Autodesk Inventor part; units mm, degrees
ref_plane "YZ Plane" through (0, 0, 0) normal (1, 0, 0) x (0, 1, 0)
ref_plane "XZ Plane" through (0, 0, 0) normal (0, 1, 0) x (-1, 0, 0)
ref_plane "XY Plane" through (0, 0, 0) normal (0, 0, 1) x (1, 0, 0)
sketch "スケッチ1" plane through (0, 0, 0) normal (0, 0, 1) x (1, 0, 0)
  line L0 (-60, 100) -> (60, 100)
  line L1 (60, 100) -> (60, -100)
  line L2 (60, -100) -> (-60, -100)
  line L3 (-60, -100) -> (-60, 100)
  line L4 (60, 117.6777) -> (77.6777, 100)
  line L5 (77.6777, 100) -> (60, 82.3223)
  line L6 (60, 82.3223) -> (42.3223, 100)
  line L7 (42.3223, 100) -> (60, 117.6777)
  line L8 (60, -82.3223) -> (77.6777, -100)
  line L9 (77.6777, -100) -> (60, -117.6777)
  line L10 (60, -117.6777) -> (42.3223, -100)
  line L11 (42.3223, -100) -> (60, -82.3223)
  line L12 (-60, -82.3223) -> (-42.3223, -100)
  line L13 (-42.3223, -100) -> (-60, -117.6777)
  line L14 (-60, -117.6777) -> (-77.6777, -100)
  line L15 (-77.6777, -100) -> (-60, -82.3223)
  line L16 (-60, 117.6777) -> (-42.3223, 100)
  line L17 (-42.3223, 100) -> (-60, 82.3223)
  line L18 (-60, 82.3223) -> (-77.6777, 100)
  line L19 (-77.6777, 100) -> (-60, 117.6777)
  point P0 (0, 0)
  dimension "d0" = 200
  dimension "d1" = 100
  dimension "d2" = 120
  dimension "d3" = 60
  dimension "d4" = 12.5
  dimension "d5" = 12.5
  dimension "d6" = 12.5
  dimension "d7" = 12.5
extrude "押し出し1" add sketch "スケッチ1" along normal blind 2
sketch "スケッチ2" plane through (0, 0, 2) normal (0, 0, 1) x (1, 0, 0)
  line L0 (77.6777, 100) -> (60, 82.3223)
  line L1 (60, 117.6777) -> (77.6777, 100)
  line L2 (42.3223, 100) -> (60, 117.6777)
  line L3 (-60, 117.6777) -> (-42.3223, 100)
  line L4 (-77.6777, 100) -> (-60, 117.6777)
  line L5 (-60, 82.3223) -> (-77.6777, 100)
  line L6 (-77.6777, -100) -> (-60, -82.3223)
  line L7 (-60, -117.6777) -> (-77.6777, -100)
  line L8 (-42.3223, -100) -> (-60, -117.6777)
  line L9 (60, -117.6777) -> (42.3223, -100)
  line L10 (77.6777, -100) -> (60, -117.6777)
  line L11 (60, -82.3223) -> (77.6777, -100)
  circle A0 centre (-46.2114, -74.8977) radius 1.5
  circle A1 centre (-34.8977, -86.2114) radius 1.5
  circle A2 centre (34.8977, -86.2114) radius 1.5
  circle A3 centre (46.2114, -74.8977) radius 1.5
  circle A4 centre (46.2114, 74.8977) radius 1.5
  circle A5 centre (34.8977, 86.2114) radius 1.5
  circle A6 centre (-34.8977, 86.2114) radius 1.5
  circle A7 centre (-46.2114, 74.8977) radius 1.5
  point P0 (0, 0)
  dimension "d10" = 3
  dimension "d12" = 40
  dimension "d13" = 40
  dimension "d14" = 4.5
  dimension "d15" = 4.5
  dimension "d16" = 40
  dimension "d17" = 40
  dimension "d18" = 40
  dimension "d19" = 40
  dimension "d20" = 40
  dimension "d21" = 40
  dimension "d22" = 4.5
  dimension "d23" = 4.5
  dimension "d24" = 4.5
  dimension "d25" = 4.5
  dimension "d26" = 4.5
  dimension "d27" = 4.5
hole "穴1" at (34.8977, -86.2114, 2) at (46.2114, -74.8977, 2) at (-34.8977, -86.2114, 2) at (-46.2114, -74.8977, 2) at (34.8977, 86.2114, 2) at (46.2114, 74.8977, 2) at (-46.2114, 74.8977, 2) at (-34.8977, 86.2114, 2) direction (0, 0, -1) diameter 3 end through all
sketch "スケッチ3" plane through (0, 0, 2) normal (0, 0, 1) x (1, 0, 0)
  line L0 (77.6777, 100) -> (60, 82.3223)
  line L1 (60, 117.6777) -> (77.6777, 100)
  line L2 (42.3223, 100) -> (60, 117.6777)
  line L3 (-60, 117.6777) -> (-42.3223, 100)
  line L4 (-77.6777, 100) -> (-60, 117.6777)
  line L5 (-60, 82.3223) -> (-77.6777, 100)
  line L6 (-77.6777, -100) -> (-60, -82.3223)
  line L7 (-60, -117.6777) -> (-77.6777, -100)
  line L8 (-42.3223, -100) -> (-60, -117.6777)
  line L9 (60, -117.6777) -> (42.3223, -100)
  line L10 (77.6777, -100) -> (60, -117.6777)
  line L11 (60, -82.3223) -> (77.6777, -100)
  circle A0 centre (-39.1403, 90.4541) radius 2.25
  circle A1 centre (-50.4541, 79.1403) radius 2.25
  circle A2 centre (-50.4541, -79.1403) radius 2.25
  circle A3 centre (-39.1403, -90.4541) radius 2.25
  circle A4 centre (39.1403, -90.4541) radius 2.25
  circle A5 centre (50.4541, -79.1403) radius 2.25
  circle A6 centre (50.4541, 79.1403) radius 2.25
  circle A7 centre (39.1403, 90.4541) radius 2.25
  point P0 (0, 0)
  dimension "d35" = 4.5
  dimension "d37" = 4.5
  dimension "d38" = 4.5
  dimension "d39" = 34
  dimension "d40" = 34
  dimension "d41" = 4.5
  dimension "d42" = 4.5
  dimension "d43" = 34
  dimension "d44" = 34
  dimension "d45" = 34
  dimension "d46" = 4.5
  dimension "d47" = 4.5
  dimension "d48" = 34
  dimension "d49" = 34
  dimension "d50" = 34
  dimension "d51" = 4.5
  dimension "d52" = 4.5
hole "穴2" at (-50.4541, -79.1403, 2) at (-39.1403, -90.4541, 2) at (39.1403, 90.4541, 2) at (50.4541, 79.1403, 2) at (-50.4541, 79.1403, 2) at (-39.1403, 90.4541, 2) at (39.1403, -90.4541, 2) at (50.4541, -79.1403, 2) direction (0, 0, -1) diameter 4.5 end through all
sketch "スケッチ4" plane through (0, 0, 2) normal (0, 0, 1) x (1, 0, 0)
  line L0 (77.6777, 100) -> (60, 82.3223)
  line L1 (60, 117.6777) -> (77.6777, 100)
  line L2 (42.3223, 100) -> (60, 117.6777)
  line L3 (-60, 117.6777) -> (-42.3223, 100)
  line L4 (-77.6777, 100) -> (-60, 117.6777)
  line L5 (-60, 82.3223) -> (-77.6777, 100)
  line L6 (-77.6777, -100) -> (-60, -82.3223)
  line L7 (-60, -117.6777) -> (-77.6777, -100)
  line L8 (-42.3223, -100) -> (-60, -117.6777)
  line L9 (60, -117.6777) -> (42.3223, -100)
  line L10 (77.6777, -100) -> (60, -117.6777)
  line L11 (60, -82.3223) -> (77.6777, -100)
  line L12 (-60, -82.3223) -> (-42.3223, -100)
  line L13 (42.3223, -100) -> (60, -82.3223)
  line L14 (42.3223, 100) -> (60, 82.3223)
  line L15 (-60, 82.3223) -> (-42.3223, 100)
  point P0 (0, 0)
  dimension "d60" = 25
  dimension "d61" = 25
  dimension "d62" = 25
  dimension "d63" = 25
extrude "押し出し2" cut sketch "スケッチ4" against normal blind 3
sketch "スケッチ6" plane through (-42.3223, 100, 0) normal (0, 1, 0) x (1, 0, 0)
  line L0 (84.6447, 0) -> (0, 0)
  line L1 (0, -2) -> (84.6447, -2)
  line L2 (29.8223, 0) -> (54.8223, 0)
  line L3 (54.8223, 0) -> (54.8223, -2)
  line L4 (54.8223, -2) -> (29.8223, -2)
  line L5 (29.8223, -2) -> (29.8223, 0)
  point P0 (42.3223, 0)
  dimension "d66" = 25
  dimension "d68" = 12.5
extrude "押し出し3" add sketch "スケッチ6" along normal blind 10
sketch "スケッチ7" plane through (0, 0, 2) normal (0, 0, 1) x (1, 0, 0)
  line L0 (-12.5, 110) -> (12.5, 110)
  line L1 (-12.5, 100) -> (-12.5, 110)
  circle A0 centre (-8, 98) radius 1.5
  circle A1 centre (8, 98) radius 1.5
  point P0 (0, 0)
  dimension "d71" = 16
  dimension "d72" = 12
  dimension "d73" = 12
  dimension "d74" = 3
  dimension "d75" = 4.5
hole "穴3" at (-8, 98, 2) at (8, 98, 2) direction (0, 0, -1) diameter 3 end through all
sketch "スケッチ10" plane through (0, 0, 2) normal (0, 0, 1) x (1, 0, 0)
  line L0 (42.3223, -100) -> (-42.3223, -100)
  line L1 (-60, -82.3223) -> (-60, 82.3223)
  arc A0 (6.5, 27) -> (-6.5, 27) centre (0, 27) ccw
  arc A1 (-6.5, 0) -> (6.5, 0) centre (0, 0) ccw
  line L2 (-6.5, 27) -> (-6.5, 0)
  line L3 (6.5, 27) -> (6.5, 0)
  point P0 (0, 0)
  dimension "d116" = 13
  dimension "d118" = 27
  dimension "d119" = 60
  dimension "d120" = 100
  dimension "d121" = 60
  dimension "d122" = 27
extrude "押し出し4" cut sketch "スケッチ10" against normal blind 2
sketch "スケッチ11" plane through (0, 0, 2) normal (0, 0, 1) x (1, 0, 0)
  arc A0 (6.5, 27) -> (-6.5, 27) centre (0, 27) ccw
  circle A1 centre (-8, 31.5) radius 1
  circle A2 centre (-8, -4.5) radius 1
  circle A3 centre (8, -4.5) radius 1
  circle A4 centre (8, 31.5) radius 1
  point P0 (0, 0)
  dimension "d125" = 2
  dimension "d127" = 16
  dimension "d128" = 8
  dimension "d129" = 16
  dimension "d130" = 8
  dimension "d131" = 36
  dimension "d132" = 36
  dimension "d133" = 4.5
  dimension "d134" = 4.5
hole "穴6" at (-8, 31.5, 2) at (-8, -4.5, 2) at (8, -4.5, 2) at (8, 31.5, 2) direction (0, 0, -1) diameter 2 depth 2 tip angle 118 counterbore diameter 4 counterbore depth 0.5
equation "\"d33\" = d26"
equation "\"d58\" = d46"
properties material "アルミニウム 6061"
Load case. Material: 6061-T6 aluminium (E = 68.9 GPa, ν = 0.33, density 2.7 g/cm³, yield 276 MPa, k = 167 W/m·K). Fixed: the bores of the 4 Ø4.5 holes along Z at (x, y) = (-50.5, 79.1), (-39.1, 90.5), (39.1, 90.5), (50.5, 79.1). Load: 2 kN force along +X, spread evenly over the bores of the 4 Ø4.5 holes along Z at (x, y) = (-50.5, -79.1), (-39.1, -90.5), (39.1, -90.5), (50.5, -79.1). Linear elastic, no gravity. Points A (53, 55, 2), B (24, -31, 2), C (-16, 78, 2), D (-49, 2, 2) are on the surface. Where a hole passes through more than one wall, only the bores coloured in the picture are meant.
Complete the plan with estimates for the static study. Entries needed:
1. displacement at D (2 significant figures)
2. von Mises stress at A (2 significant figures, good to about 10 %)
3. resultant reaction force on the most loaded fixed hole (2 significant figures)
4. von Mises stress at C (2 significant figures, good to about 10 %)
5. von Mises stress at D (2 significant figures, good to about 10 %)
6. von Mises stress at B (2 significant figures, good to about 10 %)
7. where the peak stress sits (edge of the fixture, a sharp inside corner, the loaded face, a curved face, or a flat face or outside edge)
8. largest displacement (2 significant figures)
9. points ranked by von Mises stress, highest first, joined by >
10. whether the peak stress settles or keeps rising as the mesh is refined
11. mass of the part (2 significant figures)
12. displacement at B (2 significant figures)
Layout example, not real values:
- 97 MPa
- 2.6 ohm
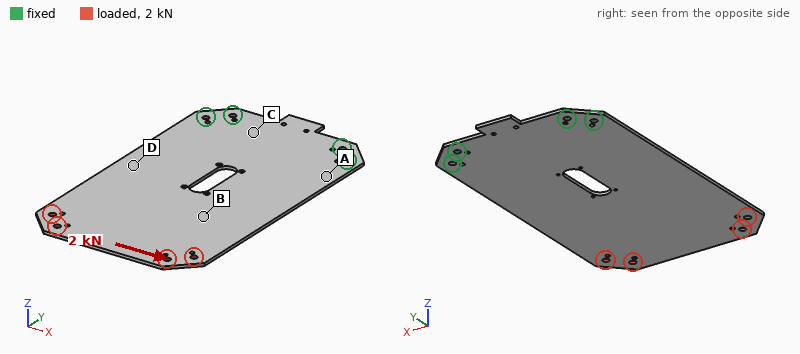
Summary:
- 0.11 mm
- 57 MPa
- 2.6 kN
- 8.3 MPa
- 29 MPa
- 21 MPa
- edge of the fixture
- 0.28 mm
- A > D > B > C
- keeps rising
- 120 g
- 0.15 mm
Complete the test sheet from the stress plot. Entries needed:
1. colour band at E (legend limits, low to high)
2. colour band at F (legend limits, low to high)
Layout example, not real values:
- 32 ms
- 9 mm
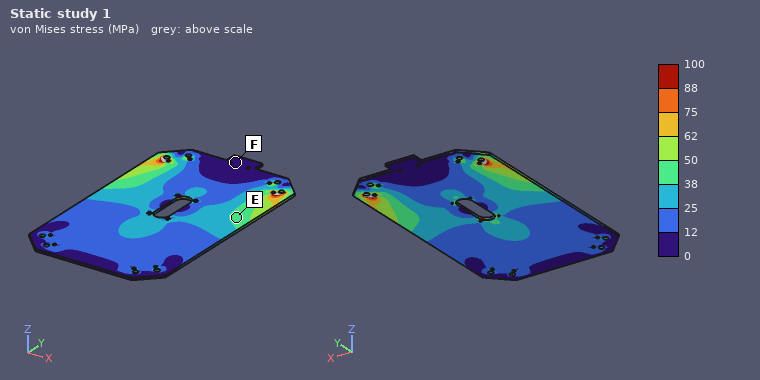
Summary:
- 38 to 50 MPa
- 0 to 12 MPa
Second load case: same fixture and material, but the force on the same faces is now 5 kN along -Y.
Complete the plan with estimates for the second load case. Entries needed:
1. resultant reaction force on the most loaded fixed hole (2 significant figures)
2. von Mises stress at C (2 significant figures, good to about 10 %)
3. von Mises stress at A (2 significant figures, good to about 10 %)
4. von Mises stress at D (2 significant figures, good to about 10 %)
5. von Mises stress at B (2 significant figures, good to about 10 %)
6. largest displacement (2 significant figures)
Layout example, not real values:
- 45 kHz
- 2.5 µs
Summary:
- 1.3 kN
- 11 MPa
- 31 MPa
- 24 MPa
- 18 MPa
- 76 µm
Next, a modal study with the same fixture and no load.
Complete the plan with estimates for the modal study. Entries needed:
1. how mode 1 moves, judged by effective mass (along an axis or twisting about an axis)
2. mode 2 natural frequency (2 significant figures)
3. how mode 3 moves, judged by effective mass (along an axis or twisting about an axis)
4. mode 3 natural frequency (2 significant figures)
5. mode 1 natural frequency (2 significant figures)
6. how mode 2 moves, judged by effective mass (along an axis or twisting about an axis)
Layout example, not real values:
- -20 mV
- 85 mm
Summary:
- along Z
- 180 Hz
- along Z
- 310 Hz
- 48 Hz
- twisting about Y
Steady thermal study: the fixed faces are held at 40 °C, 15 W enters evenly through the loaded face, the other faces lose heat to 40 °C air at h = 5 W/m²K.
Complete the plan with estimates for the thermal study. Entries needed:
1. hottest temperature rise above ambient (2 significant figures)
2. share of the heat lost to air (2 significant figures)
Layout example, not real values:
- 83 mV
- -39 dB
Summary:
- 56 K
- 39 %
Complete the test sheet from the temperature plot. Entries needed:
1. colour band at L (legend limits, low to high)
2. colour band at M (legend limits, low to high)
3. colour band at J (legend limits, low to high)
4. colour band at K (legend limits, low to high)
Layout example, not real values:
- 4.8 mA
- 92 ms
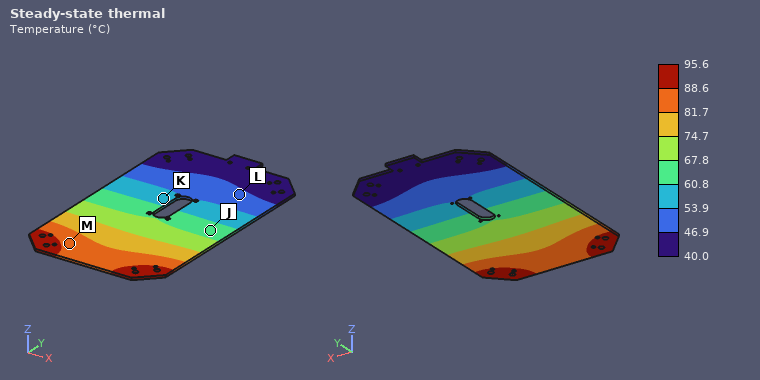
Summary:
- 46.9 to 53.9 °C
- 81.7 to 88.6 °C
- 60.8 to 67.8 °C
- 53.9 to 60.8 °C
